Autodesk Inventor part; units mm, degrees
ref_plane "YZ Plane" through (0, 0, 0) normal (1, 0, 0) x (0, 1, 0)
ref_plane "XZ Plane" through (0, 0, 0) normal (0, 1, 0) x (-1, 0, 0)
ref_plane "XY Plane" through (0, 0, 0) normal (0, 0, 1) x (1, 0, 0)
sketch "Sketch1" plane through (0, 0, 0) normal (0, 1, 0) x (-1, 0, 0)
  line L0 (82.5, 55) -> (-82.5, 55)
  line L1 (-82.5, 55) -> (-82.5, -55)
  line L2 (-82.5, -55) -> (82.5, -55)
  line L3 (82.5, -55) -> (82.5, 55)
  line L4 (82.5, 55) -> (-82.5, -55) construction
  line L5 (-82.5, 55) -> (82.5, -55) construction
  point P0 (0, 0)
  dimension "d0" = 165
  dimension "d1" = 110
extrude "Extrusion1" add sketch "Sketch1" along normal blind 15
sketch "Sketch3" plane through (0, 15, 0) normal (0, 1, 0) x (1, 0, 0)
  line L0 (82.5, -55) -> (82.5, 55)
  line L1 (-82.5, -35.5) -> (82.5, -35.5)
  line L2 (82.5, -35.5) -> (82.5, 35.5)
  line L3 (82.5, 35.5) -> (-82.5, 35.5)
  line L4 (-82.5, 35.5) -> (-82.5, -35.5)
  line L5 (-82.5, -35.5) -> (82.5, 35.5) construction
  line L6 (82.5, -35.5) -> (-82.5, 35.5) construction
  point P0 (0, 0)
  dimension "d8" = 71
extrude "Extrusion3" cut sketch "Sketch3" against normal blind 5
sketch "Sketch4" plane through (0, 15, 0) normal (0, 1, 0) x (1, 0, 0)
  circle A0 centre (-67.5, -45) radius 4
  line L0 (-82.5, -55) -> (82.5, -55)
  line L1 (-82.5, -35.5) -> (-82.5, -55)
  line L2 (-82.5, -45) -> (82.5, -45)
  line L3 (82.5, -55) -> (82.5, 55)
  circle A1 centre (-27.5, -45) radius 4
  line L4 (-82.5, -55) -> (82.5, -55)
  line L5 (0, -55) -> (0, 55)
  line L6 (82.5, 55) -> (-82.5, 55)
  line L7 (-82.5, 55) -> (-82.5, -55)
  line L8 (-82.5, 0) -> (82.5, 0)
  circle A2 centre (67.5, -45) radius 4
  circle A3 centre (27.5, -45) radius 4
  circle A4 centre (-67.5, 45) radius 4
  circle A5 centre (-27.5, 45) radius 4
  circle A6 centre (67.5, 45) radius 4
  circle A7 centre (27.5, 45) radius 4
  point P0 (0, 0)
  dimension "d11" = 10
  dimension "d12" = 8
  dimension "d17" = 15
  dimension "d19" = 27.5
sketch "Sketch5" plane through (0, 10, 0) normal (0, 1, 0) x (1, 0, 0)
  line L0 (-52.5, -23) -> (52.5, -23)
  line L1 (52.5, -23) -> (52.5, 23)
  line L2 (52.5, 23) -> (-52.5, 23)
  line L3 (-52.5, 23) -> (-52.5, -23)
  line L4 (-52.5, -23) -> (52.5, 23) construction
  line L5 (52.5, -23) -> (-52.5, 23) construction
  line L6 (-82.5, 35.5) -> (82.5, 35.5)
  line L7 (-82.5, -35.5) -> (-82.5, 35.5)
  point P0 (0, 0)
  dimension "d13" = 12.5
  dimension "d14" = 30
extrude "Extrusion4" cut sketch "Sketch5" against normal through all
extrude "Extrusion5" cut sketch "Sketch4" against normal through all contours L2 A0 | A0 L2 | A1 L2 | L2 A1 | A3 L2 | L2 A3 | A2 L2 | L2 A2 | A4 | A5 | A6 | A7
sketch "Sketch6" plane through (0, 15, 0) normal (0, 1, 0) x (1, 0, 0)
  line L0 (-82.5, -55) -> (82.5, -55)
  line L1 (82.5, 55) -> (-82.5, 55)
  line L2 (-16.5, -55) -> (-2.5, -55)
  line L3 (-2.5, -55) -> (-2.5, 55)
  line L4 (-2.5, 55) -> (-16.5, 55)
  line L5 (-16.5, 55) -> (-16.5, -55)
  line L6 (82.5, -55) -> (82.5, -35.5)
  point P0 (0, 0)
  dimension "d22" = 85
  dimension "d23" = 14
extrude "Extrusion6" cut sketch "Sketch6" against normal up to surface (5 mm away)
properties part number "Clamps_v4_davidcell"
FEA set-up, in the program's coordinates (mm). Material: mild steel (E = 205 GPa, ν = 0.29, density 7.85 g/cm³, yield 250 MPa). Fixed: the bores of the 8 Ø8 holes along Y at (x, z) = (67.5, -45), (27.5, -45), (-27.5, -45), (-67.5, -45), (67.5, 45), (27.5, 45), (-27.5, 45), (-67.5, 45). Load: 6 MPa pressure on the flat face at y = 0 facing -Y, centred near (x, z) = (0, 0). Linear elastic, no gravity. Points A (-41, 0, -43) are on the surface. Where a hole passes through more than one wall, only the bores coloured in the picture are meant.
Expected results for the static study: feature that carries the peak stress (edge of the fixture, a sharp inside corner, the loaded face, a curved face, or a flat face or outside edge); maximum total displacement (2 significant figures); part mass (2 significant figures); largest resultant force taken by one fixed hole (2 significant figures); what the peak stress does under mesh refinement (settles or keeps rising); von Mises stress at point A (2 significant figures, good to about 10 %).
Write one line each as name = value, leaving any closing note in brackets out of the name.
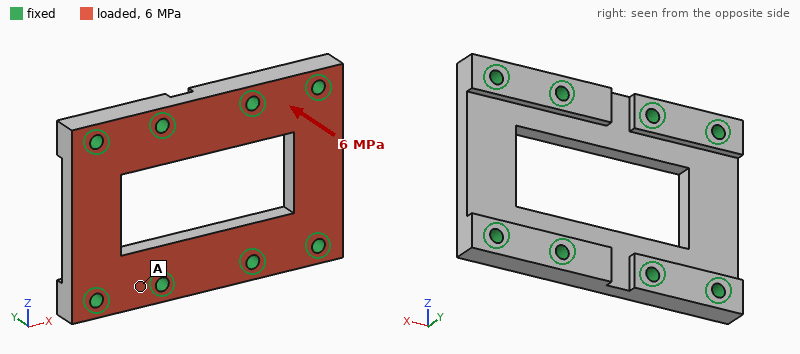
feature that carries the peak stress = edge of the fixture
maximum total displacement = 48 µm
part mass = 1.2 kg
largest resultant force taken by one fixed hole = 10 kN
what the peak stress does under mesh refinement = keeps rising
von Mises stress at point A = 31 MPa
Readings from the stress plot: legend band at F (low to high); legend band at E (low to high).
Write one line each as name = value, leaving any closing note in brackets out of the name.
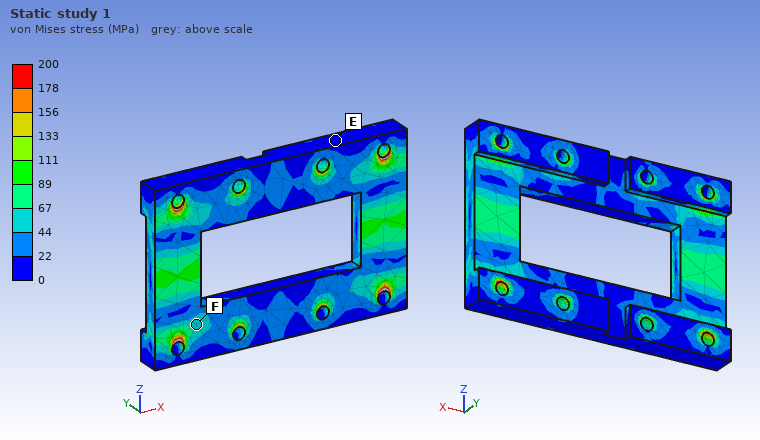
legend band at F = 44 to 67 MPa
legend band at E = 0 to 22 MPa
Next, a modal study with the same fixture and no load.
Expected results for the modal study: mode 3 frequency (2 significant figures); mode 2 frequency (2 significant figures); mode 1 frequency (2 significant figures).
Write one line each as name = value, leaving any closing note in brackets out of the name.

mode 3 frequency = 14 kHz
mode 2 frequency = 7700 Hz
mode 1 frequency = 7700 Hz
